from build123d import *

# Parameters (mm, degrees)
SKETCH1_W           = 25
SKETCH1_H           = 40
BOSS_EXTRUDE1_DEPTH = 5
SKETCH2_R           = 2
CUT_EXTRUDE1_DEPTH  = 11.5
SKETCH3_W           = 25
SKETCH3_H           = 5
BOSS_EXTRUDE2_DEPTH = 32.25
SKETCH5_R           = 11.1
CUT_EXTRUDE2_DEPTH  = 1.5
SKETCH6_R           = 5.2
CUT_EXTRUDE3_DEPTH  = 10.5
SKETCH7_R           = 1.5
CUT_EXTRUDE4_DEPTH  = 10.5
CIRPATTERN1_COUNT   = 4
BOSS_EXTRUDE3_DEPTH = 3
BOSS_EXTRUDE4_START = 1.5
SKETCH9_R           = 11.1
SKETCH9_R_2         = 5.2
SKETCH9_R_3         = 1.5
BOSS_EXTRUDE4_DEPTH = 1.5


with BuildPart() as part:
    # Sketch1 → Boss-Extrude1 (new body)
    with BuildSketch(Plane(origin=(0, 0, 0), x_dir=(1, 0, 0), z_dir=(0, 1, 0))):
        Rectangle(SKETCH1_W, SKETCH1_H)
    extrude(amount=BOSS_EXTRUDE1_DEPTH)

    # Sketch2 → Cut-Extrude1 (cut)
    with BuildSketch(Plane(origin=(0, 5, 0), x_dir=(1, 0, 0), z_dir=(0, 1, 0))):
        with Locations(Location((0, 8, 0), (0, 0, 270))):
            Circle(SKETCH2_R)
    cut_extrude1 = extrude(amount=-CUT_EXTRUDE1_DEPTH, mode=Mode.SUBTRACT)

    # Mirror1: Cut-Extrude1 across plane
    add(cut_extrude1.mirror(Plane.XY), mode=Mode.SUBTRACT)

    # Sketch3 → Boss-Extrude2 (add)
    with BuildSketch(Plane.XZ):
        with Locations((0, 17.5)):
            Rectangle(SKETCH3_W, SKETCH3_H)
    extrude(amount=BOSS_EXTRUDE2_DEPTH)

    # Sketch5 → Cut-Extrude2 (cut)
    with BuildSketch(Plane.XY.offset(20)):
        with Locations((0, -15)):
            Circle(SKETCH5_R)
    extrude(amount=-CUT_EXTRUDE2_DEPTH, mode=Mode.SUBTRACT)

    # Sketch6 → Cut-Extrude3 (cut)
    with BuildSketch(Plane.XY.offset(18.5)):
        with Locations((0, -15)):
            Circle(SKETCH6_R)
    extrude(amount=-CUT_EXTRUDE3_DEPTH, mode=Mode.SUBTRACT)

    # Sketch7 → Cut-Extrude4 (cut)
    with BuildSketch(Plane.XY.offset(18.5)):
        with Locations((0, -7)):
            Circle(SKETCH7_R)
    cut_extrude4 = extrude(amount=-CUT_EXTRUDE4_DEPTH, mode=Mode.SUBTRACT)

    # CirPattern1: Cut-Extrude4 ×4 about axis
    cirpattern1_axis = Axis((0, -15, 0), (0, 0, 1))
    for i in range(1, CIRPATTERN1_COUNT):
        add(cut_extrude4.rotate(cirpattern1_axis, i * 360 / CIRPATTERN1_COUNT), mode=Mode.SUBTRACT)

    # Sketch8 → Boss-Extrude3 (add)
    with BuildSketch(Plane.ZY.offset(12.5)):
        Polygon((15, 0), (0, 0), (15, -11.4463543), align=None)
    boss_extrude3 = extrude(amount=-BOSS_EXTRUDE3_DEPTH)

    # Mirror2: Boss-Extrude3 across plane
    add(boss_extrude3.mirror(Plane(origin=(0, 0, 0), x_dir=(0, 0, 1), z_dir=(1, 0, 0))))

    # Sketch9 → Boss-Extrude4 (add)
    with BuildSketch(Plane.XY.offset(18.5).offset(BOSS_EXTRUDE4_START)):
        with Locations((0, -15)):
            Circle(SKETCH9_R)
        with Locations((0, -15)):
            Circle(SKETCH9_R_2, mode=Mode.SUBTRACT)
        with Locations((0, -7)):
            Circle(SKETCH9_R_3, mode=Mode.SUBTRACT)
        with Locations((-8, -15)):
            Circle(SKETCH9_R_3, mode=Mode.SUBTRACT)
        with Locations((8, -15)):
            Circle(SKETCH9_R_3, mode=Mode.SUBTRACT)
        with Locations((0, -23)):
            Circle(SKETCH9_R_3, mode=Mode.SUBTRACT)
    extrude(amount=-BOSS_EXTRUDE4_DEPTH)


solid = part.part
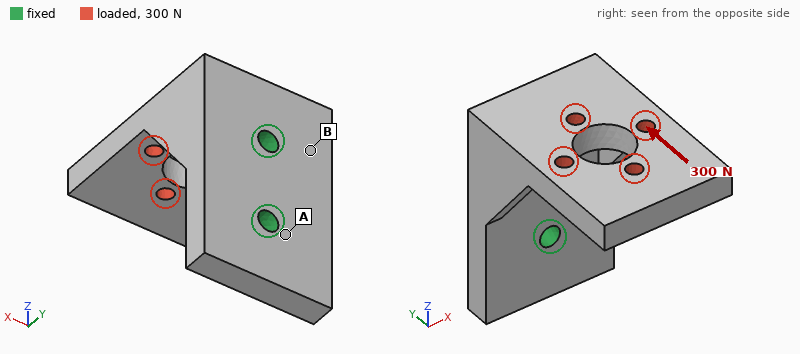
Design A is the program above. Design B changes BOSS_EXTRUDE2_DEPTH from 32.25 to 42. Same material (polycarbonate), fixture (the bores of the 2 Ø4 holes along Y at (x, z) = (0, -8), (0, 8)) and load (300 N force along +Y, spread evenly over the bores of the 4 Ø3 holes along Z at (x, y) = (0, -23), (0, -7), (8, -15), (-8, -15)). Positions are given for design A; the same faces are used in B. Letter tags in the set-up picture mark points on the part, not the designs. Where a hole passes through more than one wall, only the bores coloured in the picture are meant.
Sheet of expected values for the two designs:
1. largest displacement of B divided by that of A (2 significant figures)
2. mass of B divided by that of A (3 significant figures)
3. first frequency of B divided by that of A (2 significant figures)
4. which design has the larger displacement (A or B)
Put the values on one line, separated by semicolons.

1.2; 1.14; 0.58; B
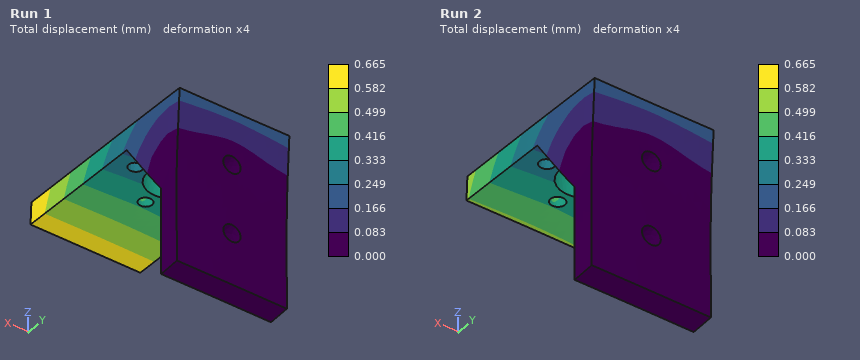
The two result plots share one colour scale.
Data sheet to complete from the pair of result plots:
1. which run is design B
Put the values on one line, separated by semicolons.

Run 1
